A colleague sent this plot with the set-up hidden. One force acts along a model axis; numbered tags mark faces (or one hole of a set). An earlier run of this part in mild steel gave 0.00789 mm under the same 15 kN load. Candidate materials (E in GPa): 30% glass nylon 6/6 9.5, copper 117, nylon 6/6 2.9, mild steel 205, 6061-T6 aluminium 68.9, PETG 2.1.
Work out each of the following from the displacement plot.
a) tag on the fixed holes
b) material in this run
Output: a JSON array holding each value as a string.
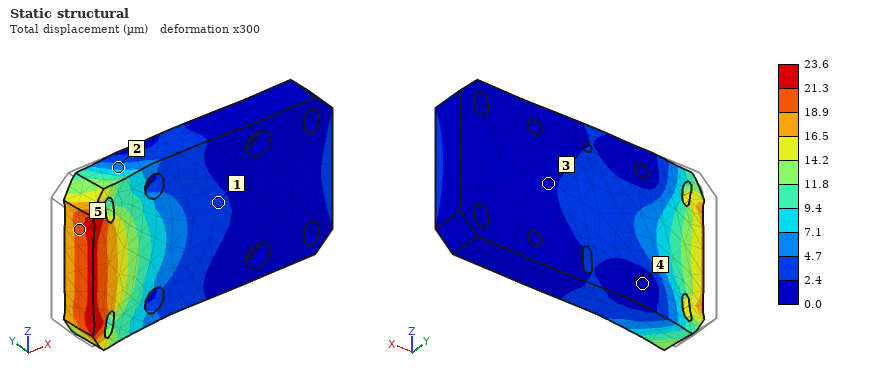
["4", "6061-T6 aluminium"]
